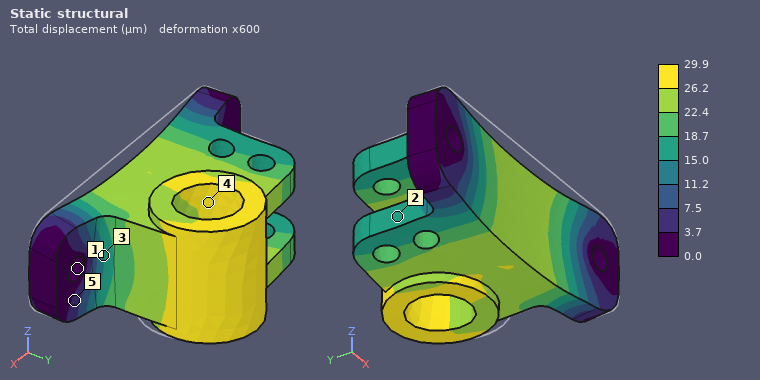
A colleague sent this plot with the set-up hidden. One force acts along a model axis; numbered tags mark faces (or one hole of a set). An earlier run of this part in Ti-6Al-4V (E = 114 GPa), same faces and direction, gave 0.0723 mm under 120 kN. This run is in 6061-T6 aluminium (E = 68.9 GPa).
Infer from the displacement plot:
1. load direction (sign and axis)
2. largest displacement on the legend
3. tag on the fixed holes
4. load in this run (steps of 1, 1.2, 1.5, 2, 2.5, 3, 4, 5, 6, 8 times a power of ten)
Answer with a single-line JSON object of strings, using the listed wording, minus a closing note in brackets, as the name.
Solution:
{"load direction": "+Y", "largest displacement on the legend": "29.9 µm", "tag on the fixed holes": "1", "load in this run": "30 kN"}
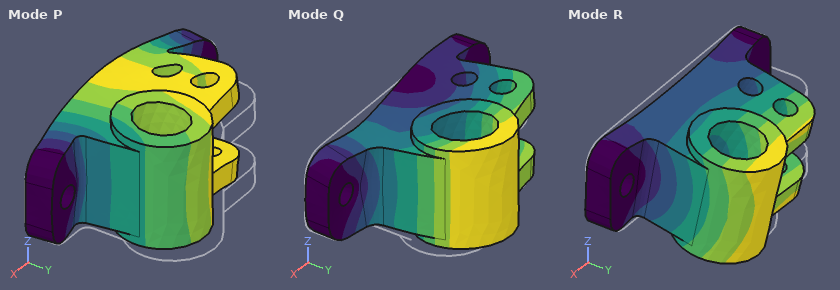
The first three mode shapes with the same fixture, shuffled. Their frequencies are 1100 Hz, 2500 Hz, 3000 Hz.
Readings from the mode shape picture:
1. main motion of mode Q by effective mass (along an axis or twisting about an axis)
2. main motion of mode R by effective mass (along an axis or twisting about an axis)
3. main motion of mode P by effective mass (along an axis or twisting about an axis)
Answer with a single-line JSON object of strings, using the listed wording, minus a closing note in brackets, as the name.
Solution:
{"main motion of mode Q by effective mass": "along X", "main motion of mode R by effective mass": "along Z", "main motion of mode P by effective mass": "along Y"}
